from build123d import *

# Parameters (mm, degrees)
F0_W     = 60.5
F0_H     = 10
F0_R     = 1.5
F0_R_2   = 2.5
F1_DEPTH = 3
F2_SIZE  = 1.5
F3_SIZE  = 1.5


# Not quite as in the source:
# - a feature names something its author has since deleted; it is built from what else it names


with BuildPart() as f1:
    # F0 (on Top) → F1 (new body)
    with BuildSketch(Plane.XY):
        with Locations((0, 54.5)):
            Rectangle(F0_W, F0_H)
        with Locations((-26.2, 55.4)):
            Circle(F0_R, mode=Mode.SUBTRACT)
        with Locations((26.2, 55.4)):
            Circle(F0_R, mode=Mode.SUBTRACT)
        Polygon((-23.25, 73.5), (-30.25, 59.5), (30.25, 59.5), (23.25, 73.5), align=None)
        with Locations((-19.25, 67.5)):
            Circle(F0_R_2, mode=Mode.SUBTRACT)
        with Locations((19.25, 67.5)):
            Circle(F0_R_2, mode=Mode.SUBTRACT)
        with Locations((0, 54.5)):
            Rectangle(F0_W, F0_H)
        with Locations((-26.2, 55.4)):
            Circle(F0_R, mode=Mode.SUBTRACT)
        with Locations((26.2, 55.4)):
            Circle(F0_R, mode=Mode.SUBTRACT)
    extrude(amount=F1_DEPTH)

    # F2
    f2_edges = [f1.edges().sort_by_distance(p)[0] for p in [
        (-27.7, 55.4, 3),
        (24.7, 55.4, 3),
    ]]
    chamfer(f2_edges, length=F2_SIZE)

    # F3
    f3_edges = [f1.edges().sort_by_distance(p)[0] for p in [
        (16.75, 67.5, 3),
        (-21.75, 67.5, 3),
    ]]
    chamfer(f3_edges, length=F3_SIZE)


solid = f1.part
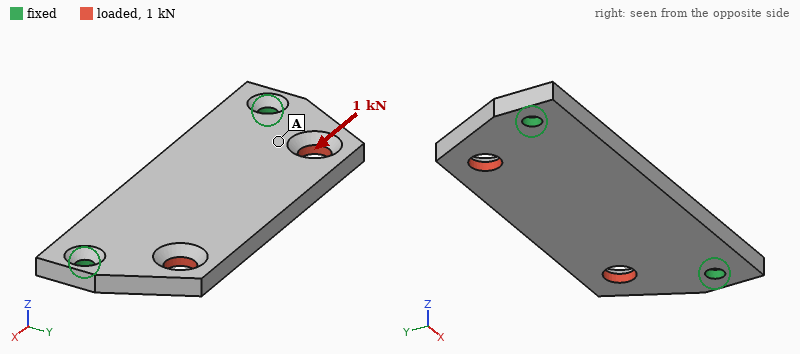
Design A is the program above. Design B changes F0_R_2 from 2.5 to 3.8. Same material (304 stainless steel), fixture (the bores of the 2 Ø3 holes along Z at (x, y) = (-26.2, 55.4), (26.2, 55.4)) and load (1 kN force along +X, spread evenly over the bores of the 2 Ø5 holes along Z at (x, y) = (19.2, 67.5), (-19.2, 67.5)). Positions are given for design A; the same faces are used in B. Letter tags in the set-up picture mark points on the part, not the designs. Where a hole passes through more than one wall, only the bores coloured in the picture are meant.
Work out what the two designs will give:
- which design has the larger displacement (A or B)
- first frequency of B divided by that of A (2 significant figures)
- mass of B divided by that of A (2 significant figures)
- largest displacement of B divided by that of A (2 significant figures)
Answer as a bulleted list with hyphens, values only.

- B
- 1.0
- 0.95
- 1.2
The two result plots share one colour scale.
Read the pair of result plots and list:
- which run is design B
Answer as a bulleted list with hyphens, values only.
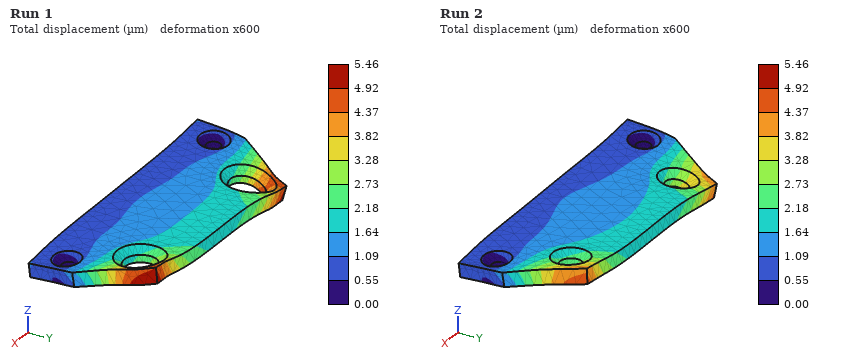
- Run 1
